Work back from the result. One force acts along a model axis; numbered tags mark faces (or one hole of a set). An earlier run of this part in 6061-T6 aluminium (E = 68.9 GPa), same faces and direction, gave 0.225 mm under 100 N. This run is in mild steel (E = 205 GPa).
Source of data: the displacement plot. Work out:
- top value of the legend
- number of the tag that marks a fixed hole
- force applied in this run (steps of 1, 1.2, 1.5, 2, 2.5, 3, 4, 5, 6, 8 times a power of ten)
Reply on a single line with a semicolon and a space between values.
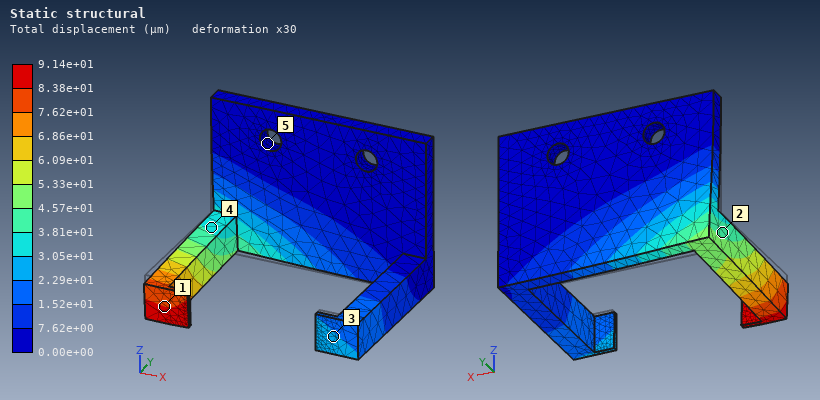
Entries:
9.14e+01 µm; 5; 120 N
